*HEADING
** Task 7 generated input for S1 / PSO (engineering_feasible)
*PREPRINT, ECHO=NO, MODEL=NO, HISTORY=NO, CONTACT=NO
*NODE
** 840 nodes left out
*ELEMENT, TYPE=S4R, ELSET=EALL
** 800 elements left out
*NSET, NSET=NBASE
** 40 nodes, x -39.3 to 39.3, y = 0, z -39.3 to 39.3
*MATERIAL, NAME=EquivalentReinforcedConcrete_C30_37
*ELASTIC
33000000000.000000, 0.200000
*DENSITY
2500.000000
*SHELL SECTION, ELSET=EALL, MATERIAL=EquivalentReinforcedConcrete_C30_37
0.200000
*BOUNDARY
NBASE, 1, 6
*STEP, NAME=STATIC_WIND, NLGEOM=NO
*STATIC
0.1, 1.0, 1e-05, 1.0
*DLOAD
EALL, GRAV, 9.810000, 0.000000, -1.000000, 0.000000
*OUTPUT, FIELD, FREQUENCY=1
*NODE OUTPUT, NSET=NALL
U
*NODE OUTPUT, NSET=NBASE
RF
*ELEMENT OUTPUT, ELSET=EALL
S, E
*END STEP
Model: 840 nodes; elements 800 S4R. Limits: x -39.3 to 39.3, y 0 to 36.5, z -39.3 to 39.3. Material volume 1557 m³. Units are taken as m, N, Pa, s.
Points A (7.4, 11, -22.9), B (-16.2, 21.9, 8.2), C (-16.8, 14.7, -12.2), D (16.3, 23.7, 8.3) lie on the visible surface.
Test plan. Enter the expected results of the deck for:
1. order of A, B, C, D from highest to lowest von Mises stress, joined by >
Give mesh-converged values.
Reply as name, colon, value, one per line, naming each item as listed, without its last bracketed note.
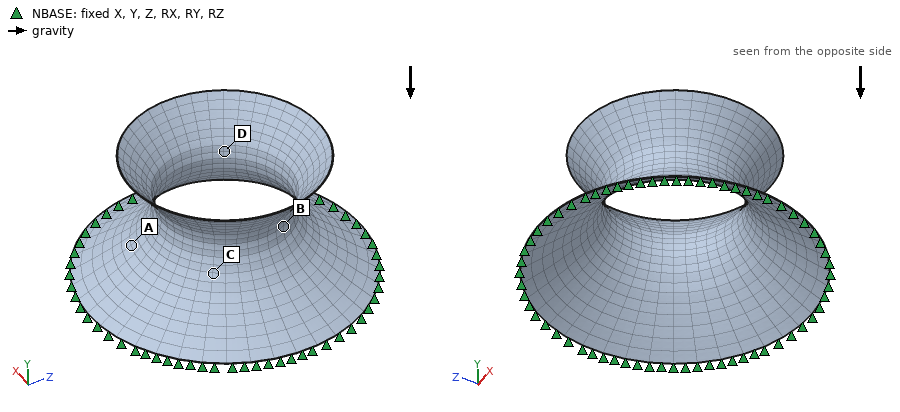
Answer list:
order of A, B, C, D from highest to lowest von Mises stress, joined by >: A > C > B > D
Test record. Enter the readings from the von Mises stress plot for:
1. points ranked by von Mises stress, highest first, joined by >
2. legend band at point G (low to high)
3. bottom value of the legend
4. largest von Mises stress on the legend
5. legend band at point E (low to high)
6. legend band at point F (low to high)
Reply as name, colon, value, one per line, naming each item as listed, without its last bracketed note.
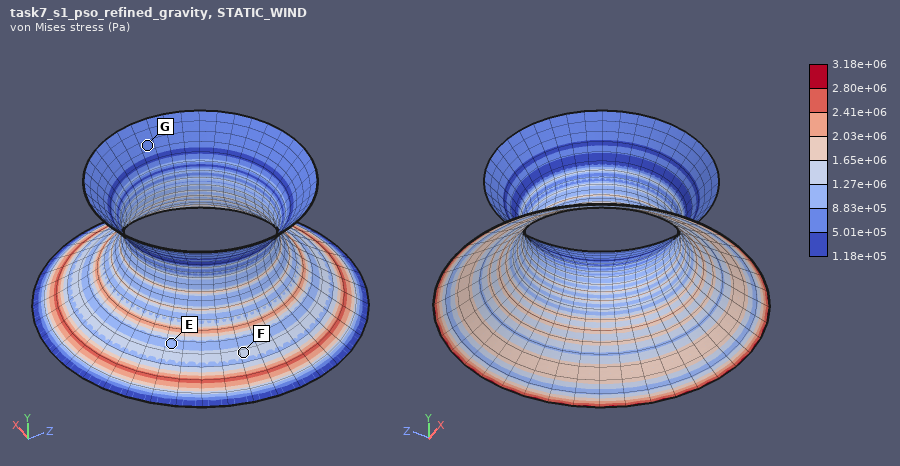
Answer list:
points ranked by von Mises stress, highest first, joined by >: F > E > G
legend band at point G: 5.01e+05 to 8.83e+05 Pa
bottom value of the legend: 1.18e+05 Pa
largest von Mises stress on the legend: 3.18e+06 Pa
legend band at point E: 8.83e+05 to 1.27e+06 Pa
legend band at point F: 1.27e+06 to 1.65e+06 Pa
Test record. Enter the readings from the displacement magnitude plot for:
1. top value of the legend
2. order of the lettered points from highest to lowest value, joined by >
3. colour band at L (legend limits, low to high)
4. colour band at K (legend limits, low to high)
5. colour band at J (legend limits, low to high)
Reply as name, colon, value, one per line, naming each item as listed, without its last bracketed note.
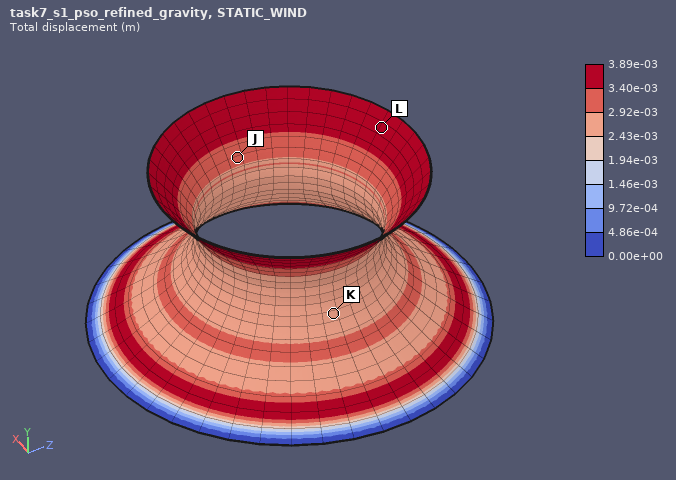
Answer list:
top value of the legend: 3.89e-03 m
order of the lettered points from highest to lowest value, joined by >: L > J > K
colour band at L: 3.40e-03 to 3.89e-03 m
colour band at K: 2.43e-03 to 2.92e-03 m
colour band at J: 2.92e-03 to 3.40e-03 m
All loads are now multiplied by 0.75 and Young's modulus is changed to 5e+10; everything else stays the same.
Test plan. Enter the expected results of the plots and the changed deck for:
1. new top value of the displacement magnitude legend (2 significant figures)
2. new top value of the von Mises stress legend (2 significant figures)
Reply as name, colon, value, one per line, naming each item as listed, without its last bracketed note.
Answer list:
new top value of the displacement magnitude legend: 0.0019 m
new top value of the von Mises stress legend: 2.4e+06 Pa
